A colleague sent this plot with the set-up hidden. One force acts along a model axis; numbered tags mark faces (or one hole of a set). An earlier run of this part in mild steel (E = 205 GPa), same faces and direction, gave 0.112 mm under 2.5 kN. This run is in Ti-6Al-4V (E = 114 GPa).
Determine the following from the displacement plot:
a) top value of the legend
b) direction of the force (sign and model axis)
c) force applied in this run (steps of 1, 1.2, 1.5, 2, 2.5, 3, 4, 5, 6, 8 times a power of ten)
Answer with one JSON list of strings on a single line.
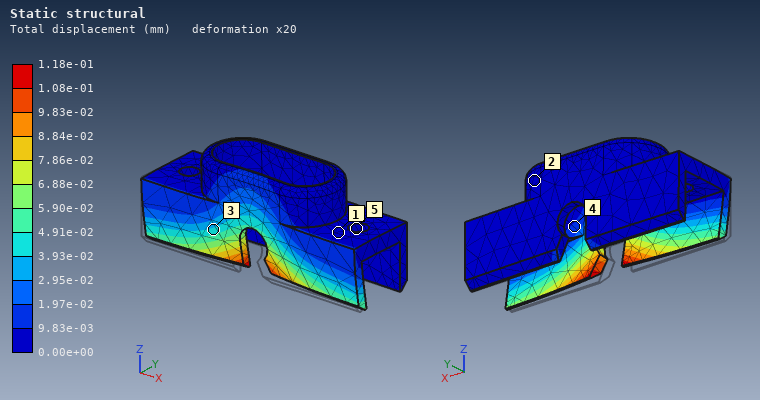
["1.18e-01 mm", "+Y", "1.5 kN"]
